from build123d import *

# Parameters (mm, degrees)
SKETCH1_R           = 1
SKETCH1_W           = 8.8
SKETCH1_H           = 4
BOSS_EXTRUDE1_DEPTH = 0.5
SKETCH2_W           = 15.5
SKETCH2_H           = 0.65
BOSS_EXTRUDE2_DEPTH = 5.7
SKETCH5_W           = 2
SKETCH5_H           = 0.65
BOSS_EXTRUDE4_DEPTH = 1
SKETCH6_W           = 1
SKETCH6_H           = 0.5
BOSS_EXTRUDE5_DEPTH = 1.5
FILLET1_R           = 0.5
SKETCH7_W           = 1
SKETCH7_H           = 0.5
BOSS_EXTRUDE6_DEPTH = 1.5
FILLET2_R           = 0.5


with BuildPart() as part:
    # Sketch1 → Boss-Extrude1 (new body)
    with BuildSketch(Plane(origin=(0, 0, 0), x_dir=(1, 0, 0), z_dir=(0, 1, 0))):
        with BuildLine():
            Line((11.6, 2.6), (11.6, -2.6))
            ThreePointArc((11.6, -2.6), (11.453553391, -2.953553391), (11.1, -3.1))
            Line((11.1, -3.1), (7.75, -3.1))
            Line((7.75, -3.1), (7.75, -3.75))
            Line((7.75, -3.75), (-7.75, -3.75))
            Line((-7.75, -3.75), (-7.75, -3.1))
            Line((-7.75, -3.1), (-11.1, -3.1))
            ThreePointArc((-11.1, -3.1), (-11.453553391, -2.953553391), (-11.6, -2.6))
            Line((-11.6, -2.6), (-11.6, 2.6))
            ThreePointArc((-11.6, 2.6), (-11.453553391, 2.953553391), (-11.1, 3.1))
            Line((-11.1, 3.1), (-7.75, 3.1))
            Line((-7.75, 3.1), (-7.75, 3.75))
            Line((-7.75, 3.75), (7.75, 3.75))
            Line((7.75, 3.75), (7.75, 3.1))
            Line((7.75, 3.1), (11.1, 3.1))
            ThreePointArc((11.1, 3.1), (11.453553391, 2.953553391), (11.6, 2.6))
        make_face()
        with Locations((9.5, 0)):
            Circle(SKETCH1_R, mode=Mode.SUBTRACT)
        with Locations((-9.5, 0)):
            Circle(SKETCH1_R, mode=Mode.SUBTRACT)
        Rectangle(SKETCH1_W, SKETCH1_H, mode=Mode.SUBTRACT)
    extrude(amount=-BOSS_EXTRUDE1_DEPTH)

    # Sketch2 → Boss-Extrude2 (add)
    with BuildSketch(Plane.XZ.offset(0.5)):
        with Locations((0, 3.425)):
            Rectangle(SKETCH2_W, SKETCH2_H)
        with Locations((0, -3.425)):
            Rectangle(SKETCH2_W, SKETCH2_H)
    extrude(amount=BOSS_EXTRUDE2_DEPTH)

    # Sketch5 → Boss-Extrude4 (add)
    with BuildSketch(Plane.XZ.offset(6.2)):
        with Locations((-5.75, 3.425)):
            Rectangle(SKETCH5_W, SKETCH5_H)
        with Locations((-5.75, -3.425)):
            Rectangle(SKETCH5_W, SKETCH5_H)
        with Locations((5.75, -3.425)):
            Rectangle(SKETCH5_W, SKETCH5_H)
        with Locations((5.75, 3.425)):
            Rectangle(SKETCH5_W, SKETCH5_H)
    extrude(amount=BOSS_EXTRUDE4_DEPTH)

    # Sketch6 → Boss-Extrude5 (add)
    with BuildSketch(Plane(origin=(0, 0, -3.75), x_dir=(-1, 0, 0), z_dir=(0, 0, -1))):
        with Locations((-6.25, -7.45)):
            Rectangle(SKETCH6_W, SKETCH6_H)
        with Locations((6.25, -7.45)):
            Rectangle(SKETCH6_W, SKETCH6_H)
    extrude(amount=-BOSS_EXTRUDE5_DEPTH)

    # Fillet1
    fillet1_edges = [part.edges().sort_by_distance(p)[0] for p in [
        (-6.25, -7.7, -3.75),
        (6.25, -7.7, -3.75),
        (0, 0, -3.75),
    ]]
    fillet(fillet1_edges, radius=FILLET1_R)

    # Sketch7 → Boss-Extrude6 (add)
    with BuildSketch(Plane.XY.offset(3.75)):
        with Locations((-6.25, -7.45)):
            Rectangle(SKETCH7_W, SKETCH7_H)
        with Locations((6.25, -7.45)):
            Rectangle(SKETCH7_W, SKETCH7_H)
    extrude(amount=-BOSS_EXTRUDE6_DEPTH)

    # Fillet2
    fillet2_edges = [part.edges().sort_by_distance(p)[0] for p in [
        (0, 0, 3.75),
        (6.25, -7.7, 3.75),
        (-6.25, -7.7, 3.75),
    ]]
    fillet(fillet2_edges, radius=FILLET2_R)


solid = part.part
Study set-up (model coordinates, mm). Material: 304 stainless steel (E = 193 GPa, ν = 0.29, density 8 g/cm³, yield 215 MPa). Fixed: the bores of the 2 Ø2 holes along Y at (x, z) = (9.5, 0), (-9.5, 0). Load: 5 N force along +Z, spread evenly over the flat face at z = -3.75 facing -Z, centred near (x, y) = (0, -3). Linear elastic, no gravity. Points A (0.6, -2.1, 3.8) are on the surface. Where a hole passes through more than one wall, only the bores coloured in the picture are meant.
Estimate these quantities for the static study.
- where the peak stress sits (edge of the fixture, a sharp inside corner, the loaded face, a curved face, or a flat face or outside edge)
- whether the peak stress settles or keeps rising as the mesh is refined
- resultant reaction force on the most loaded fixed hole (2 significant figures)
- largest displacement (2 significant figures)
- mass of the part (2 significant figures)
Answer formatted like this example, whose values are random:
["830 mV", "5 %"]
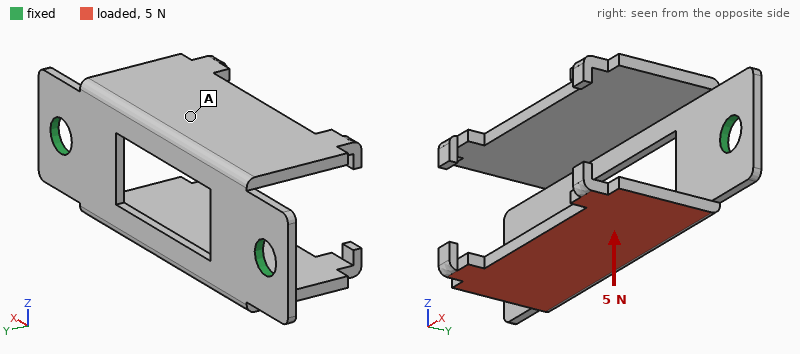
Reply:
["a sharp inside corner", "keeps rising", "2.6 N", "22 µm", "1.5 g"]
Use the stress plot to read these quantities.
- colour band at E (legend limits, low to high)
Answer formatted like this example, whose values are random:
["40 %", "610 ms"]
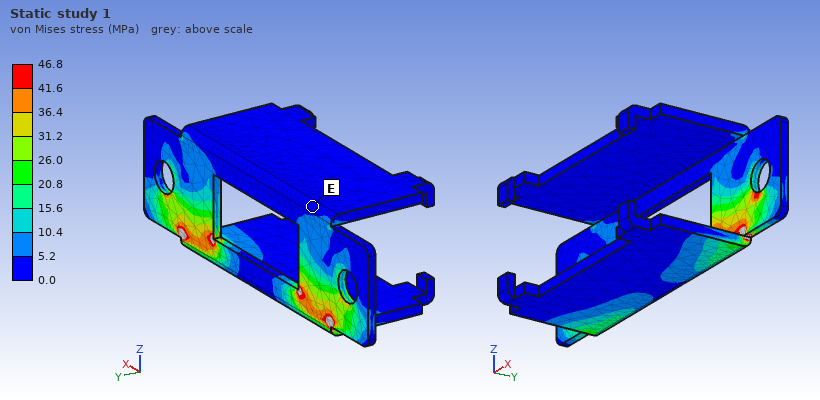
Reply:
["0.0 to 5.2 MPa"]
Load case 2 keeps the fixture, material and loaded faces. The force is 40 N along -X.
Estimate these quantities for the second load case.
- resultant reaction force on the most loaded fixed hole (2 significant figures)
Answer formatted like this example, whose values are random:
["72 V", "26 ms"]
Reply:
["22 N"]
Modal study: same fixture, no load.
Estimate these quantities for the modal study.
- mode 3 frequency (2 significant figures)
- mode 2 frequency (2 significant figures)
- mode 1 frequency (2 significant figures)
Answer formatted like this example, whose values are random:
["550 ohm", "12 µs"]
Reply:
["10 kHz", "4200 Hz", "4200 Hz"]
